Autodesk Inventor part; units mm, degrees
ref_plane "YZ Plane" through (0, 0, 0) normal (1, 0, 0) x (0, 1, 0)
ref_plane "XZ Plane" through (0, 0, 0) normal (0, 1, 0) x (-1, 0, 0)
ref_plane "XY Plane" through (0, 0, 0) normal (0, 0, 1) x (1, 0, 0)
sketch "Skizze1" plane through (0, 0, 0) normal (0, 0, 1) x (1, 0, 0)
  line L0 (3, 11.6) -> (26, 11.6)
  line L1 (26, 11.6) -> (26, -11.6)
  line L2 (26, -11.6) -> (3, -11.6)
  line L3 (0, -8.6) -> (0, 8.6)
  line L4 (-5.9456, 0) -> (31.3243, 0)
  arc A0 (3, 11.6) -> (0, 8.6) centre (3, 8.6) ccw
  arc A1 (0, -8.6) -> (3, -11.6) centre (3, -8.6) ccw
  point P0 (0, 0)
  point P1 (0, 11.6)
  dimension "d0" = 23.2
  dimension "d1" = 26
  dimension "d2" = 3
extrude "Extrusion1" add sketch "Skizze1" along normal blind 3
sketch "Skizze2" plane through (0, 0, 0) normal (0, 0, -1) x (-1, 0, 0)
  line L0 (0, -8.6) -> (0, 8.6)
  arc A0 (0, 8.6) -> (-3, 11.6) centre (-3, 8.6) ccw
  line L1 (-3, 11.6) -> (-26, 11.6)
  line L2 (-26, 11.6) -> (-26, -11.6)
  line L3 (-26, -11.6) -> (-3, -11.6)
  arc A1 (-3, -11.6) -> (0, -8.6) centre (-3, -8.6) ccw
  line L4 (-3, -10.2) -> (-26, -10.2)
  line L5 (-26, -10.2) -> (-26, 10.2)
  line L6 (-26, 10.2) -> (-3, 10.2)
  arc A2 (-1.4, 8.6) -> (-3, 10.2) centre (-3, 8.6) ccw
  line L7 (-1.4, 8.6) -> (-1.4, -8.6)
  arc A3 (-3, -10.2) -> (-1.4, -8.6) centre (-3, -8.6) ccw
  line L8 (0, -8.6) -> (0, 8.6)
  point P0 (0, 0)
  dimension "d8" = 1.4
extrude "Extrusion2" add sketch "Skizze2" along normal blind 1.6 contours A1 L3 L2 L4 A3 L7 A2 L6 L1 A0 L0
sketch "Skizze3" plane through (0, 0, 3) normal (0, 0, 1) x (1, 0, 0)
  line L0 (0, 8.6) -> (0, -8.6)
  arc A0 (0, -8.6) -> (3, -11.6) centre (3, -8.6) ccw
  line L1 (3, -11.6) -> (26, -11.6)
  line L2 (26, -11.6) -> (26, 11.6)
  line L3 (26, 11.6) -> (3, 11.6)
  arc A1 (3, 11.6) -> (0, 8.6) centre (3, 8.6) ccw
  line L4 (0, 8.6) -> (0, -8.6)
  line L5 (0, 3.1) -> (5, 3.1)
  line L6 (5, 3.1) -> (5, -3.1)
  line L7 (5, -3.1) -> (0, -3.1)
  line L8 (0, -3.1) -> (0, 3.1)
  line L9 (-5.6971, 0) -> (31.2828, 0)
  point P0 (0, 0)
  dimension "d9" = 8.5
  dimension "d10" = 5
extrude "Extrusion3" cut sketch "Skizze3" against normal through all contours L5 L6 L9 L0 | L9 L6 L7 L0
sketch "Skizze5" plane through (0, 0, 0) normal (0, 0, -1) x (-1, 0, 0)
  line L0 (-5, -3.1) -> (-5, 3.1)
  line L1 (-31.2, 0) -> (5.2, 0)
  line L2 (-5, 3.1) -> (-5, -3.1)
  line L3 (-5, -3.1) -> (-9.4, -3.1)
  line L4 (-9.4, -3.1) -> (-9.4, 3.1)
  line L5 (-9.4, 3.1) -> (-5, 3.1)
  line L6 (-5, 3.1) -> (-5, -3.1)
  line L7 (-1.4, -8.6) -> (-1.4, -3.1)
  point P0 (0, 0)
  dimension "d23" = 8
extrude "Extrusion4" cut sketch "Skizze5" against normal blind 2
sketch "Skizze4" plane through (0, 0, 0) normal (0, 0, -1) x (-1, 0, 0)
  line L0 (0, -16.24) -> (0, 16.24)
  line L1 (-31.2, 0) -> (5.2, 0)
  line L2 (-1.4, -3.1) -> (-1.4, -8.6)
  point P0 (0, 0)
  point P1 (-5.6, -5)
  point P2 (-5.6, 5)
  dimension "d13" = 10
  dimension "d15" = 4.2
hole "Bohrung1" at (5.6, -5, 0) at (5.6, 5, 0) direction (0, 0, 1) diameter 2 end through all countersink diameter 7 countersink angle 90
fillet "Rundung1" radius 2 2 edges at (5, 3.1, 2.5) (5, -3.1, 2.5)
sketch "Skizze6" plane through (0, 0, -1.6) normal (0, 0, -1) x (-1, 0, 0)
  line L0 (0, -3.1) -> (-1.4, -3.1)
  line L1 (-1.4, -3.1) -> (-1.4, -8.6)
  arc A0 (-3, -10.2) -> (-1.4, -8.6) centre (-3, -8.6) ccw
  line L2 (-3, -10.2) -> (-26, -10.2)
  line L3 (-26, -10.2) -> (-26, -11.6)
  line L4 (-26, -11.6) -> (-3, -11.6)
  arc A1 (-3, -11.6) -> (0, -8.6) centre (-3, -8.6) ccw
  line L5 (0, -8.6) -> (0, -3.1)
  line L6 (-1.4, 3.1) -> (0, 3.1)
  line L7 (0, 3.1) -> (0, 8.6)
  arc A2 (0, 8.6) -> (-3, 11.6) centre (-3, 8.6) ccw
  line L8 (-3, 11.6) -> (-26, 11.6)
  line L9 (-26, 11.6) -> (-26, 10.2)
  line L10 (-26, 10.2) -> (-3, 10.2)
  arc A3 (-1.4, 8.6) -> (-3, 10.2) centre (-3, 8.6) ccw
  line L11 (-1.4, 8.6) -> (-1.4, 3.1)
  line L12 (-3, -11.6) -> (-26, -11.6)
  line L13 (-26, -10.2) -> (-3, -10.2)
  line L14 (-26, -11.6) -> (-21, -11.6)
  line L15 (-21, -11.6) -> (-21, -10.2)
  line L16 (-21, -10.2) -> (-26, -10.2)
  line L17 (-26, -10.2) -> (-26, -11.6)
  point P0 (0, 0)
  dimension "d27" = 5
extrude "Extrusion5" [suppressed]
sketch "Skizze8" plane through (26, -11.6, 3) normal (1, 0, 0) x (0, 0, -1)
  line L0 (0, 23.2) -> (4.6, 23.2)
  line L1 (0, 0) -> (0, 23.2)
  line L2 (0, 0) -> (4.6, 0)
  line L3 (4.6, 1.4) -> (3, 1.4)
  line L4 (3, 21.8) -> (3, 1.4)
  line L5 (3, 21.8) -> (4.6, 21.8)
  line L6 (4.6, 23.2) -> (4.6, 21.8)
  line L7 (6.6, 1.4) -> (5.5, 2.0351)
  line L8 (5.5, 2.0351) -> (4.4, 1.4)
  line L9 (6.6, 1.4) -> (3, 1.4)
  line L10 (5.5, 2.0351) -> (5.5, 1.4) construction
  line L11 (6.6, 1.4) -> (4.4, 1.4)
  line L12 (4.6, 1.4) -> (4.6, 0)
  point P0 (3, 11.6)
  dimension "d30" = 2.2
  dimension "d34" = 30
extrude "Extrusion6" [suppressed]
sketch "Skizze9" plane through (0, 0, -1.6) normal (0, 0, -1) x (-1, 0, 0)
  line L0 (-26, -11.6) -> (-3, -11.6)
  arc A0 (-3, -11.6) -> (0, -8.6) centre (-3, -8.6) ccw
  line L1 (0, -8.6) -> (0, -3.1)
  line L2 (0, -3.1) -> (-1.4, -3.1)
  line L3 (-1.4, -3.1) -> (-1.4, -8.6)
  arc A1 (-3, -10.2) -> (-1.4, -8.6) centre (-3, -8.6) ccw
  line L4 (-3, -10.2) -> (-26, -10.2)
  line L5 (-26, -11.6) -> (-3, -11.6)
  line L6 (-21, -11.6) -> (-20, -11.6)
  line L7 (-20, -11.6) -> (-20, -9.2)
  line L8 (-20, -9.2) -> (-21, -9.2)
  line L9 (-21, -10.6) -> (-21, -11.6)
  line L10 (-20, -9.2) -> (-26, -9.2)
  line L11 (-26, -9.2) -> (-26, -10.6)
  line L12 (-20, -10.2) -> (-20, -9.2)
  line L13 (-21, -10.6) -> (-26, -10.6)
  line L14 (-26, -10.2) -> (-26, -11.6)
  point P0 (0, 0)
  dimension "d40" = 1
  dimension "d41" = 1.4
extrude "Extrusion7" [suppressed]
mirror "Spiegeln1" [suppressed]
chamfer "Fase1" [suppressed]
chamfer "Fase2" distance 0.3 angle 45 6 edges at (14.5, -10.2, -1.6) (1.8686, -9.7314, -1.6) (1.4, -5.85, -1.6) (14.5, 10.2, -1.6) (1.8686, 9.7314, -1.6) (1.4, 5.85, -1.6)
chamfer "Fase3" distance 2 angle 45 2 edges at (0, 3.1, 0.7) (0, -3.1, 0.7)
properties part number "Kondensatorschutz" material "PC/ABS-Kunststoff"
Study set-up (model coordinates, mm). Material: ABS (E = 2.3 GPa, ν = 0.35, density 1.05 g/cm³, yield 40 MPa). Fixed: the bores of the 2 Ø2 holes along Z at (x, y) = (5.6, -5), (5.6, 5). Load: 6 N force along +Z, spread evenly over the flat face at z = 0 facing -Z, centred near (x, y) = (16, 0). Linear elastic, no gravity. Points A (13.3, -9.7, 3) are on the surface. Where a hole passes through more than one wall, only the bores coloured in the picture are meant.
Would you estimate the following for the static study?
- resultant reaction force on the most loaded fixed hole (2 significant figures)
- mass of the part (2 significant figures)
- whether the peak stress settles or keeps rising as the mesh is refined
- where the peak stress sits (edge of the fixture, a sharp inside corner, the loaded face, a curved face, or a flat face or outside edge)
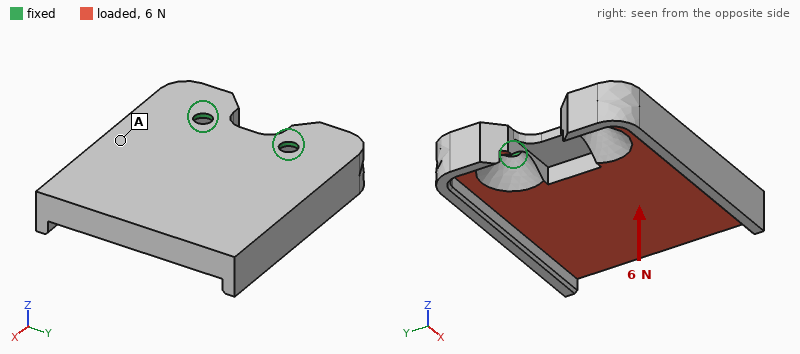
3.4 N
1.8 g
keeps rising
edge of the fixture
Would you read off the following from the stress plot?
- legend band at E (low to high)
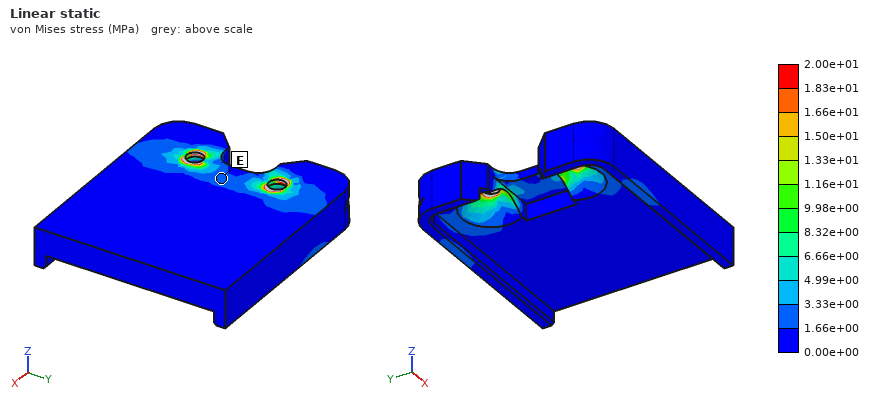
1.66e+00 to 3.33e+00 MPa
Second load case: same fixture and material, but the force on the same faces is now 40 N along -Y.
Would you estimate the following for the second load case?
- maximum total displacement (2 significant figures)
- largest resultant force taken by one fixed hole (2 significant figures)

100 µm
44 N
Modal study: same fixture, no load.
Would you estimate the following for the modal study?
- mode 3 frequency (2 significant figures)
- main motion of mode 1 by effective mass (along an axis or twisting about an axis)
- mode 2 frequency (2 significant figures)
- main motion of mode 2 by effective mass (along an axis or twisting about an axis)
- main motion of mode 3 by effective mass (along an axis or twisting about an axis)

3500 Hz
along Z
1900 Hz
twisting about X
along Y
